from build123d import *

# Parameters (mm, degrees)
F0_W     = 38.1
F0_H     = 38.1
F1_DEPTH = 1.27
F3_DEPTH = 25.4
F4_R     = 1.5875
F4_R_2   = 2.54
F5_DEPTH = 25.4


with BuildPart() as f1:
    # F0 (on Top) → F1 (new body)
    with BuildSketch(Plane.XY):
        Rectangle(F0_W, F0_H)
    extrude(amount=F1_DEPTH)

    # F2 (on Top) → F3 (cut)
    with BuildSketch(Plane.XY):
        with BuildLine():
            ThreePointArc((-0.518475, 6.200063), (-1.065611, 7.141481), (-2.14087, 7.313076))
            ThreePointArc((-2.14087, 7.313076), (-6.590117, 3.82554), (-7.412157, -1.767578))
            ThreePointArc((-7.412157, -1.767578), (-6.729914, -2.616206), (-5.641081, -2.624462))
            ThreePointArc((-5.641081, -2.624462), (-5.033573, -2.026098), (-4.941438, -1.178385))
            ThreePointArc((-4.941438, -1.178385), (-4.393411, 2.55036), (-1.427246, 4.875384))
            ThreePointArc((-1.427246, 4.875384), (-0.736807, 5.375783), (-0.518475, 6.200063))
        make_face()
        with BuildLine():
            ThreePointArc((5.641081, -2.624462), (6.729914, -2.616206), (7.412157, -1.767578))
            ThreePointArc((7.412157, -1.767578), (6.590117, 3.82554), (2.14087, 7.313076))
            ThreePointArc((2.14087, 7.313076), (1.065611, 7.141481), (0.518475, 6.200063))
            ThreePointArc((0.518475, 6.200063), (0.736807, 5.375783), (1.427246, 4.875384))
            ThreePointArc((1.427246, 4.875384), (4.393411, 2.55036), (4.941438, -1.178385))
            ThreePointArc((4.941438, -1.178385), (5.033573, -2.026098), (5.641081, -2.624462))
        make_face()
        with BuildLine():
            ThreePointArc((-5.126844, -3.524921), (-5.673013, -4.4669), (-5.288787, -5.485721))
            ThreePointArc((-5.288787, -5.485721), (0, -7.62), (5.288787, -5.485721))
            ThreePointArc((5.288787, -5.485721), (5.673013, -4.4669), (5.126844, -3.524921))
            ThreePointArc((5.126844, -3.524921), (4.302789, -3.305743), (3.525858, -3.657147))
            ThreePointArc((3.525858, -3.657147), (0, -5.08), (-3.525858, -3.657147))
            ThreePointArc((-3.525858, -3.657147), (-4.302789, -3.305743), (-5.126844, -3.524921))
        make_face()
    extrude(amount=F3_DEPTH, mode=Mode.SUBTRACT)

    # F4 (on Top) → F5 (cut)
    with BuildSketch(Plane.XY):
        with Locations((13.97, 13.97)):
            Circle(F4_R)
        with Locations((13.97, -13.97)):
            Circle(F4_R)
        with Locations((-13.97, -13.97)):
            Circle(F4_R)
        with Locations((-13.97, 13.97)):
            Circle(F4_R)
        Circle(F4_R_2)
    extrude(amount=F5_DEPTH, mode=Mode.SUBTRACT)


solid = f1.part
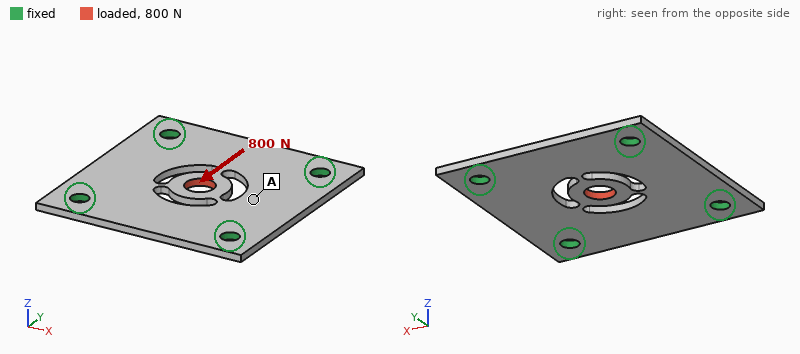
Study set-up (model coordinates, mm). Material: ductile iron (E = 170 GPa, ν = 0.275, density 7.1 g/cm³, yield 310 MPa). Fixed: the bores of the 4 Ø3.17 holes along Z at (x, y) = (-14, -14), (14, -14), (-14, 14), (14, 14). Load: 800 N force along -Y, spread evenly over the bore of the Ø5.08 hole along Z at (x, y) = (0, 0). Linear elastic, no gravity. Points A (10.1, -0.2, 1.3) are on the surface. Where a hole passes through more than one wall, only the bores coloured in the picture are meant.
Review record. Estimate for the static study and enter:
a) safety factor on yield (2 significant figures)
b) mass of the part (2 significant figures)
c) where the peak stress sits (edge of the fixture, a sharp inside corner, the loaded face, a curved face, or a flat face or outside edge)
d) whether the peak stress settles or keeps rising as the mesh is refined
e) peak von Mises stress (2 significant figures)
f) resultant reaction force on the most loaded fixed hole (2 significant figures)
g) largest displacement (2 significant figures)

0.59
12 g
a curved face
settles
530 MPa
240 N
18 µm
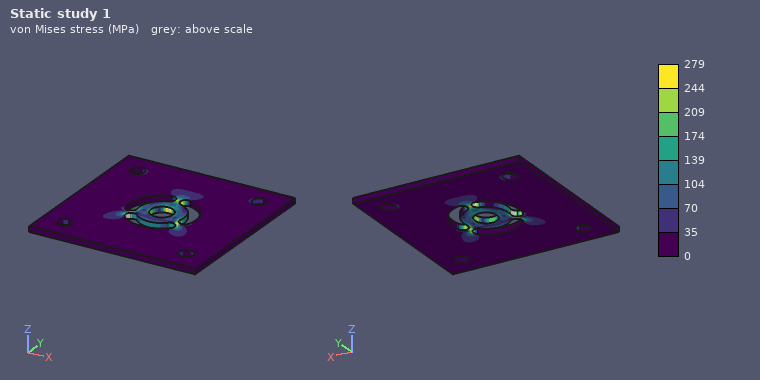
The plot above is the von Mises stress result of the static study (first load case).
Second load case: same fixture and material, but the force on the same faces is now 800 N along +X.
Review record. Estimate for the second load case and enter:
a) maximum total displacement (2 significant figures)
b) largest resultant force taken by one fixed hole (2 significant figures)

17 µm
270 N
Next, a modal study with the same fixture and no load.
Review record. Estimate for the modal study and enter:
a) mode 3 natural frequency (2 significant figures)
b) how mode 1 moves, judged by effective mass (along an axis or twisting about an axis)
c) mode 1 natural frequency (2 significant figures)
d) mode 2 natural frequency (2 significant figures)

9500 Hz
along Z
6500 Hz
9500 Hz
